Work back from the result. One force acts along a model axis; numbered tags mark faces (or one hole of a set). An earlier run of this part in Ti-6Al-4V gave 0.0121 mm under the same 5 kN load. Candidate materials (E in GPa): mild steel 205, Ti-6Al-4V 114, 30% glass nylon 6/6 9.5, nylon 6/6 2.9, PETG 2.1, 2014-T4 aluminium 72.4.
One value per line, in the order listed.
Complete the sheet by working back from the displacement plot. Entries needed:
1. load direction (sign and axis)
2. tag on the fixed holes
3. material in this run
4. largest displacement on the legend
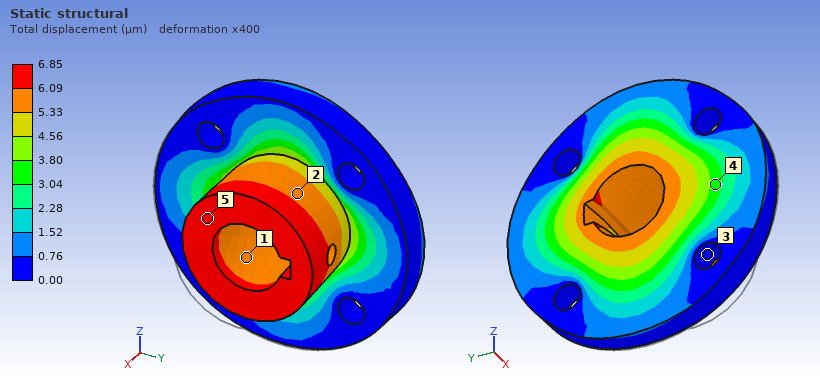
-X
3
mild steel
6.85 µm
